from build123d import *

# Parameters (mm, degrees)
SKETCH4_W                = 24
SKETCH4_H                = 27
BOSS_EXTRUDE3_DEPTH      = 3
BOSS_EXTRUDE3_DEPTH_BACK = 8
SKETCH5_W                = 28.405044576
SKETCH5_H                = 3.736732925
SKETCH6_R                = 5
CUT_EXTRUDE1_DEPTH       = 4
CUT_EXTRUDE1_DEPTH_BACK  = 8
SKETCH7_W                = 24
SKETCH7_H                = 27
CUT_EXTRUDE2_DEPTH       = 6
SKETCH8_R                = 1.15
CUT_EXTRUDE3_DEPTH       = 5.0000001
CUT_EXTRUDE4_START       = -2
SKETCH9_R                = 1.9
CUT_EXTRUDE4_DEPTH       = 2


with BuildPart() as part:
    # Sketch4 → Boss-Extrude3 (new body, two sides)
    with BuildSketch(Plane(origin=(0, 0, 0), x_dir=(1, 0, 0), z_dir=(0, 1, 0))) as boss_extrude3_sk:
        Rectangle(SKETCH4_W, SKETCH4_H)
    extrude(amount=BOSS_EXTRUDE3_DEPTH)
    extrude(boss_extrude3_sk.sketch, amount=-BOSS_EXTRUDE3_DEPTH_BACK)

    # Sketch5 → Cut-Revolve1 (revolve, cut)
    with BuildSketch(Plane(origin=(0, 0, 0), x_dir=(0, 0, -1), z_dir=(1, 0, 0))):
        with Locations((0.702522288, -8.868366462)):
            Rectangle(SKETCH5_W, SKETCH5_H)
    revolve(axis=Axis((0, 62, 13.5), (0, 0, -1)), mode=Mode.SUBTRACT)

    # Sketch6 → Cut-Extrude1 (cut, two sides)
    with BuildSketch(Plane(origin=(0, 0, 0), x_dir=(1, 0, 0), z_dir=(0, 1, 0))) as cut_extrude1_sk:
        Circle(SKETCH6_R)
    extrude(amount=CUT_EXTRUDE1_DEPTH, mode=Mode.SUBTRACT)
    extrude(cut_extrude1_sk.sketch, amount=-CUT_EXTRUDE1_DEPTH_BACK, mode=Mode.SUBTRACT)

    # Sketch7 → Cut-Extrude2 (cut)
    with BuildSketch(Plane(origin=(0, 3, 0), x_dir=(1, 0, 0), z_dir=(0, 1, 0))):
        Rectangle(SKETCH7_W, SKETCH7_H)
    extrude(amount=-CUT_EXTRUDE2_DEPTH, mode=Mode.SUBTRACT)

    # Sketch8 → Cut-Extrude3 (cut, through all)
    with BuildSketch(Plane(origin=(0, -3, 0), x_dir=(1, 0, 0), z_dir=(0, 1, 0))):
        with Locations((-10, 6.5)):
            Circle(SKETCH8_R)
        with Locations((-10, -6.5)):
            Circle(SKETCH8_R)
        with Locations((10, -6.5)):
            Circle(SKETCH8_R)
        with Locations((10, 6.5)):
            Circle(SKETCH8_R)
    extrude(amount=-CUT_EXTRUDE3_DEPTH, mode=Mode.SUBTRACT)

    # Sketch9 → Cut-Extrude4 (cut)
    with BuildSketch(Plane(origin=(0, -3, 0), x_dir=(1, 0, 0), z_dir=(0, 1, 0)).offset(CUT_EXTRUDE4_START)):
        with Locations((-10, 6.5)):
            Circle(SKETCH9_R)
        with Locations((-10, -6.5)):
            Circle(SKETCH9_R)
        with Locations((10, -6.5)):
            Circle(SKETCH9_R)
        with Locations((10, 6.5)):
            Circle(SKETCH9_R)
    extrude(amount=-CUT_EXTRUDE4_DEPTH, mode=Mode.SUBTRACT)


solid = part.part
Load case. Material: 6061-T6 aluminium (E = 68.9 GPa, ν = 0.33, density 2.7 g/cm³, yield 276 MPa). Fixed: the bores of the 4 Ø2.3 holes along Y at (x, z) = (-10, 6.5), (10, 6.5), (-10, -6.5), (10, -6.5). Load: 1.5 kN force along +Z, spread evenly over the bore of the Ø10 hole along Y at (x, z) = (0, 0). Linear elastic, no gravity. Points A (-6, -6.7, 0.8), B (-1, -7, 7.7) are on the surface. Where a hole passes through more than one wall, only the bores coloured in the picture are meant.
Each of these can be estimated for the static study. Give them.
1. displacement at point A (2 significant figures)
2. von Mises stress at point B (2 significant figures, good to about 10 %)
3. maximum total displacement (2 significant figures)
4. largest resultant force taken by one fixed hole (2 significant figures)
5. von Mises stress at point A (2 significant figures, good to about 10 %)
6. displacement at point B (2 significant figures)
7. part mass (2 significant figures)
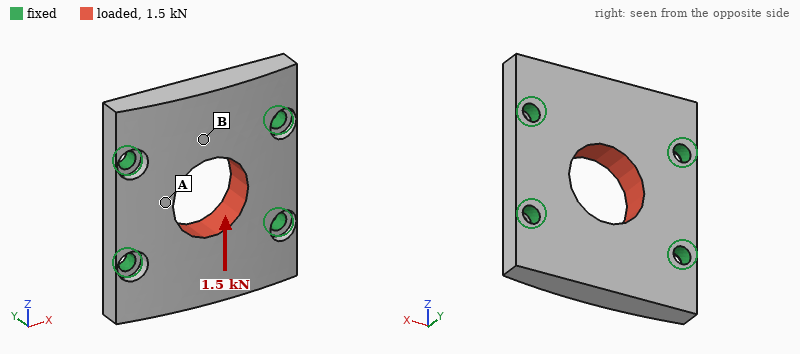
2.4 µm
8.7 MPa
4.7 µm
380 N
25 MPa
4.2 µm
5.3 g
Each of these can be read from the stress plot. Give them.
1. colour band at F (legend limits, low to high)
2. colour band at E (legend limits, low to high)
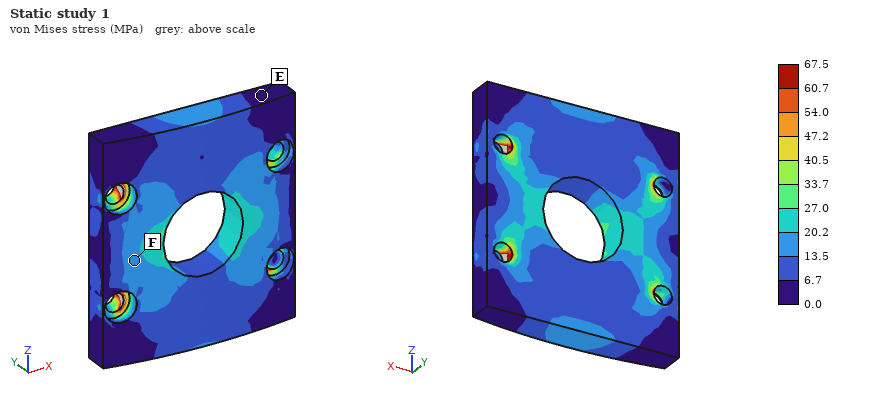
13.5 to 20.2 MPa
0.0 to 6.7 MPa
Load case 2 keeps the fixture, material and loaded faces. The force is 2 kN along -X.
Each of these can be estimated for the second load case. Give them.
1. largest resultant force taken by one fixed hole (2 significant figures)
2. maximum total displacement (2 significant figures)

520 N
4.8 µm
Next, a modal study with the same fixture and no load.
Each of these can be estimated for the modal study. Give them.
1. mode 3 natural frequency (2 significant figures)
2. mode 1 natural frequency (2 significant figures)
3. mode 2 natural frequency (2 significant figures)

39 kHz
25 kHz
25 kHz
